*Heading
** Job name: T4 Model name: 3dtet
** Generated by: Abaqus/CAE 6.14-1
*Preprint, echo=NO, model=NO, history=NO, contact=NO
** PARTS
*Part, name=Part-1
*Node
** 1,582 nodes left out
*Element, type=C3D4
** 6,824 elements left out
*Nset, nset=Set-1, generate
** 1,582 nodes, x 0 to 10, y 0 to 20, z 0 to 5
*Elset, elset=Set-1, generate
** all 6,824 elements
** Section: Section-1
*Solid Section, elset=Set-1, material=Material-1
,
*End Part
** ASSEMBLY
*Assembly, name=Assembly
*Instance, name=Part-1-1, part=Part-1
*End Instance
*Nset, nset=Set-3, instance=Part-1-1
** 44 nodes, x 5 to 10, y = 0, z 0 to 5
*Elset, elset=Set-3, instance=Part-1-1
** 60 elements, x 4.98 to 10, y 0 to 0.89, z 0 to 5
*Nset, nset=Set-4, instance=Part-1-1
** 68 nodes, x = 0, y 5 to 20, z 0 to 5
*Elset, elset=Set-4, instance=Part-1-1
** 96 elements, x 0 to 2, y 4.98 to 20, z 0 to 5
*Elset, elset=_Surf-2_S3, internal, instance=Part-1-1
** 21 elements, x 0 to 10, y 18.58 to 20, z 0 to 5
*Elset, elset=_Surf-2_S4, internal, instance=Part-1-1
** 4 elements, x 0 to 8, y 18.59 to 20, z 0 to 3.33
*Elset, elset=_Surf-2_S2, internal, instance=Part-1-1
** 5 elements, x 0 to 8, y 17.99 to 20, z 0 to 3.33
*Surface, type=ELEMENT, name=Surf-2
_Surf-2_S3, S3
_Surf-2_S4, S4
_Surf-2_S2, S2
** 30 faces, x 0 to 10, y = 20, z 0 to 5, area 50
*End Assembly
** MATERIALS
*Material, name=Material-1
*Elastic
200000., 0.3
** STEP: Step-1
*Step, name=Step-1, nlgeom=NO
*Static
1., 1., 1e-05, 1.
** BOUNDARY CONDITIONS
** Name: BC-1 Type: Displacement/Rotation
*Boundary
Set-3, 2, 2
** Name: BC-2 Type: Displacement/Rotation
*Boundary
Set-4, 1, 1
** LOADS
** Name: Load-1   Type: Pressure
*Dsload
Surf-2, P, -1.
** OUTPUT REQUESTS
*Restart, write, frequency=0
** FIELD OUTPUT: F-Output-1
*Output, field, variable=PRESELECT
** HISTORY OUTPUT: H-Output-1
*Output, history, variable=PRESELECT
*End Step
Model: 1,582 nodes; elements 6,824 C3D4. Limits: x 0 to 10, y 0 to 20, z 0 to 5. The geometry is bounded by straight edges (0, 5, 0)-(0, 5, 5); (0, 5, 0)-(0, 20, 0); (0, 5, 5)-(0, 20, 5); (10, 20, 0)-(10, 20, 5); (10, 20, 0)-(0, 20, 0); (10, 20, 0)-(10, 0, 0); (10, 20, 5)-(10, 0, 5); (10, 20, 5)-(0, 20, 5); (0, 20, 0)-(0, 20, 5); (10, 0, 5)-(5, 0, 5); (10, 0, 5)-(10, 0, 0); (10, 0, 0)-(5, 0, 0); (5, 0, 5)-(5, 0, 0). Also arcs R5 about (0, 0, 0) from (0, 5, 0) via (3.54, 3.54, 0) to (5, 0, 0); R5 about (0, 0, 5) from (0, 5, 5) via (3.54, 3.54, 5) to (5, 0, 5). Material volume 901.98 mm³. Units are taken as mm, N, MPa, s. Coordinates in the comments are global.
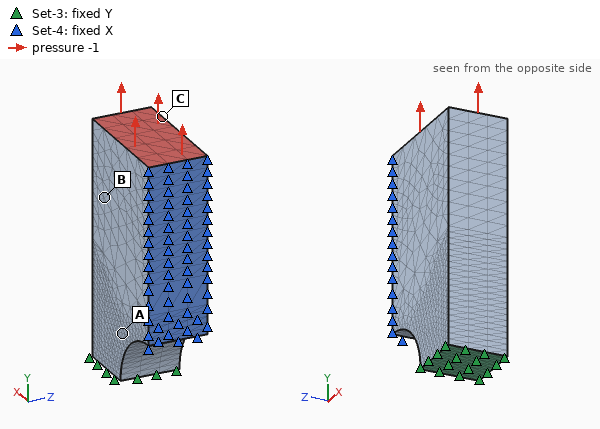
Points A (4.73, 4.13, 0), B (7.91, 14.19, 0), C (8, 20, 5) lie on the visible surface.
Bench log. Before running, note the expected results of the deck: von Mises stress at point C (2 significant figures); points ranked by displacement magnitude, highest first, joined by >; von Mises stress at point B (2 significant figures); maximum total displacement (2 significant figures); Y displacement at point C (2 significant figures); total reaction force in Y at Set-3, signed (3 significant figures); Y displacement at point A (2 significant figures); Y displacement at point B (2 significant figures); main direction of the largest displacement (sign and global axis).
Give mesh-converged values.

1.0 MPa
C > B > A
1.2 MPa
1.5e-04 mm
1.4e-04 mm
-50.0 N
5.8e-05 mm
1.1e-04 mm
+Y
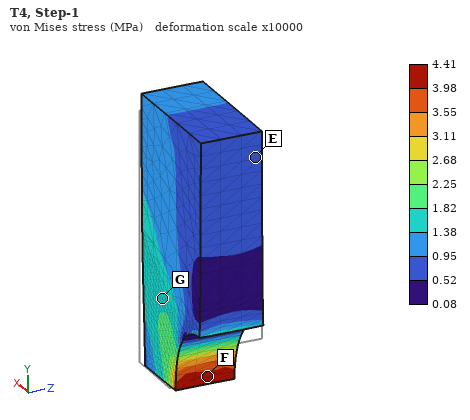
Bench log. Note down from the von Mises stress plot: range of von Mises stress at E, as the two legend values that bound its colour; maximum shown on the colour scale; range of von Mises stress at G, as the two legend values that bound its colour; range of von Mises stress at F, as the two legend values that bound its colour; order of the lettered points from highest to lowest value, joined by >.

0.52 to 0.95 MPa
4.41 MPa
1.38 to 1.82 MPa
3.98 to 4.41 MPa
F > G > E
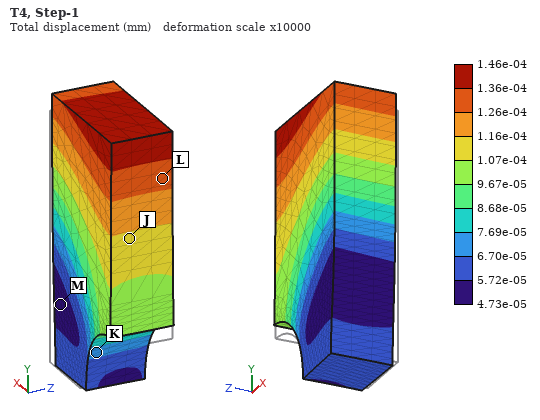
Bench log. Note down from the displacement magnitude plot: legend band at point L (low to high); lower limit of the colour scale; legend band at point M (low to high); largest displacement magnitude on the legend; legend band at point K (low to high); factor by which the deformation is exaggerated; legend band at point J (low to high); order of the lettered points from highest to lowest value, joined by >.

1.26e-04 to 1.36e-04 mm
4.73e-05 mm
4.73e-05 to 5.72e-05 mm
1.46e-04 mm
6.70e-05 to 7.69e-05 mm
10000
1.07e-04 to 1.16e-04 mm
L > J > K > M
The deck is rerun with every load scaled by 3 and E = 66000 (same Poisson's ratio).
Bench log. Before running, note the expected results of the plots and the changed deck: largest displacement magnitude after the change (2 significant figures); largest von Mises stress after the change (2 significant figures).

0.0013 mm
13 MPa
